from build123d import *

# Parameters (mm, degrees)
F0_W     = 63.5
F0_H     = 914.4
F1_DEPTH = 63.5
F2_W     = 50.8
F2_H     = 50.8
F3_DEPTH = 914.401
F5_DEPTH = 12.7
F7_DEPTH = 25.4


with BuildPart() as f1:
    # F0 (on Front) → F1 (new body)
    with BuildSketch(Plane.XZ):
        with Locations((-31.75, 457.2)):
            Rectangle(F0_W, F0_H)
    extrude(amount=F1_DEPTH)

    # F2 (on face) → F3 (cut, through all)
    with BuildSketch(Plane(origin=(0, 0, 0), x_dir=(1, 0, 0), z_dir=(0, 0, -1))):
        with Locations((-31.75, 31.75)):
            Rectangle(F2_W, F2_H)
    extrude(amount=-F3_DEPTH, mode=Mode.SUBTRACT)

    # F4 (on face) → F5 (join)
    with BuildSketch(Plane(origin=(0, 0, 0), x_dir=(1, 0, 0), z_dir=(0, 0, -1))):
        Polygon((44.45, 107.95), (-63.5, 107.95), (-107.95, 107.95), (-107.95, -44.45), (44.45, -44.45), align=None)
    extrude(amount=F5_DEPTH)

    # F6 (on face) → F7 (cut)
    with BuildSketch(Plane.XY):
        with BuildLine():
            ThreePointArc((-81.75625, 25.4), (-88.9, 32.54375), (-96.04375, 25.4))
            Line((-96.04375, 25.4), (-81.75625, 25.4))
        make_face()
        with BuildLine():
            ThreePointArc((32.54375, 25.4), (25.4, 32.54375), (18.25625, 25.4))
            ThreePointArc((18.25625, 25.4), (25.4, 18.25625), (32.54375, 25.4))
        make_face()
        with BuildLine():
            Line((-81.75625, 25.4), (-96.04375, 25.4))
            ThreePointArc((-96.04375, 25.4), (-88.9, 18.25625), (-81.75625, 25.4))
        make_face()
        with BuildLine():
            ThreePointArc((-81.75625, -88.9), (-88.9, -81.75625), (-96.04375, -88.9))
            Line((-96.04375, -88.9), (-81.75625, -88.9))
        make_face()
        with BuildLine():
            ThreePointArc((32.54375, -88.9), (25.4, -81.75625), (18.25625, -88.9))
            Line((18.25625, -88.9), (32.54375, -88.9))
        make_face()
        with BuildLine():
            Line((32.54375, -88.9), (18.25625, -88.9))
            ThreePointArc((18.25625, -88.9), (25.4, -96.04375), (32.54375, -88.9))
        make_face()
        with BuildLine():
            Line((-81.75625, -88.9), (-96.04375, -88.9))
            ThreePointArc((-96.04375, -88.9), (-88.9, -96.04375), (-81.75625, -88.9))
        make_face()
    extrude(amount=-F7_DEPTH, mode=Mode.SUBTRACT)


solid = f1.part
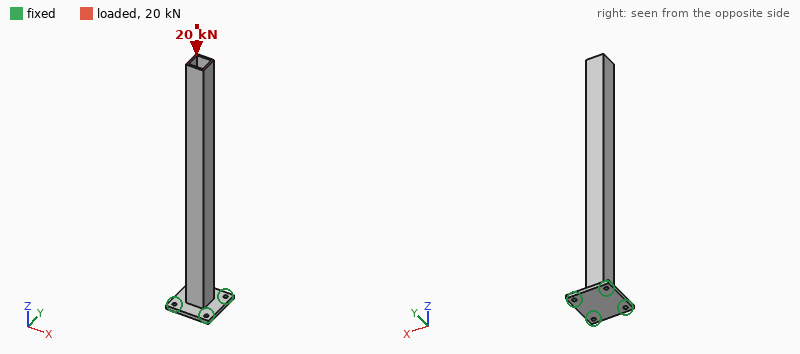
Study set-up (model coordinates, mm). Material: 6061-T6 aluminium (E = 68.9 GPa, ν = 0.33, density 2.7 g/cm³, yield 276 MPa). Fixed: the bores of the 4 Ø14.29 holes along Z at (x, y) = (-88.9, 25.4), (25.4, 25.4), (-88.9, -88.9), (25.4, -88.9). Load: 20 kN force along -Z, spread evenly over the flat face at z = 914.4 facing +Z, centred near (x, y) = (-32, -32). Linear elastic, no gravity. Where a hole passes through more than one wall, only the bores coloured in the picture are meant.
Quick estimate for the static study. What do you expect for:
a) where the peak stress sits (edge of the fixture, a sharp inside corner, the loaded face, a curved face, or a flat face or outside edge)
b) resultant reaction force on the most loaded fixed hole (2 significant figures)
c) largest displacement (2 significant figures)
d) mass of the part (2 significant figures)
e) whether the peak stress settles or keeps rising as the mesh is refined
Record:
edge of the fixture
5.1 kN
0.26 mm
4.4 kg
keeps rising
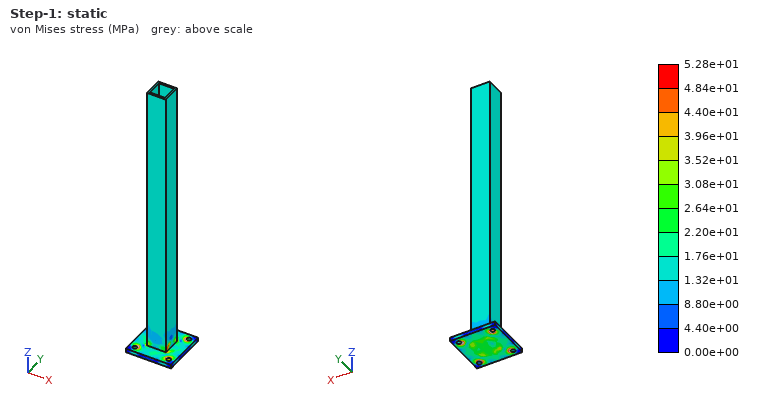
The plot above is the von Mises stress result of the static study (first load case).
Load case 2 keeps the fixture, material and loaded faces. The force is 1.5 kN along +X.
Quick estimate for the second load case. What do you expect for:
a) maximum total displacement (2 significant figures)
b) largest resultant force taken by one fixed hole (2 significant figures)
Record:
9.5 mm
7.3 kN
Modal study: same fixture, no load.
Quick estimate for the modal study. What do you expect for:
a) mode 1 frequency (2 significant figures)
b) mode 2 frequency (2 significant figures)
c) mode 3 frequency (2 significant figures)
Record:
65 Hz
65 Hz
410 Hz
